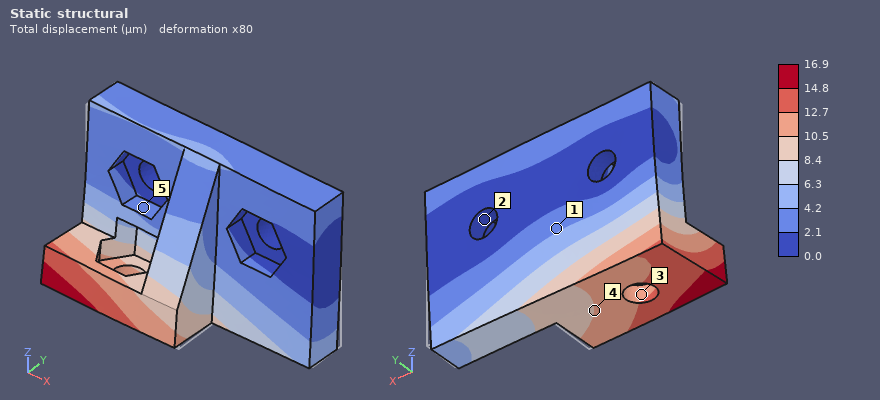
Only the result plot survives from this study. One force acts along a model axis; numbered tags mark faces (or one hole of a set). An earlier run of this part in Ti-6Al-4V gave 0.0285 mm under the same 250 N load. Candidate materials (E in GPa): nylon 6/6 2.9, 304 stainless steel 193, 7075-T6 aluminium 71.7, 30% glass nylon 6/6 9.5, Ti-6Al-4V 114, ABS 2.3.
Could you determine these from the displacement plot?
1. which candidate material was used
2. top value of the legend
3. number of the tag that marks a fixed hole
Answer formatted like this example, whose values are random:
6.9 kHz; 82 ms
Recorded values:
304 stainless steel; 16.9 µm; 2
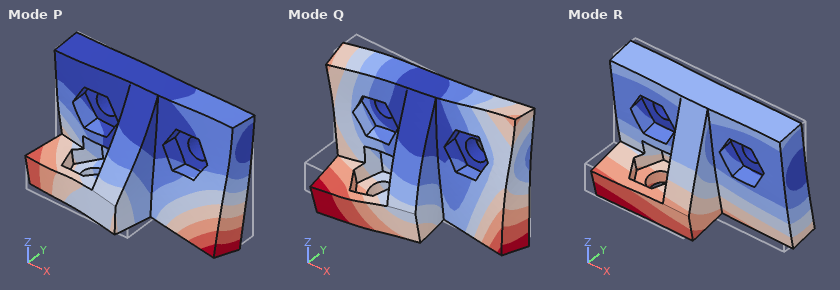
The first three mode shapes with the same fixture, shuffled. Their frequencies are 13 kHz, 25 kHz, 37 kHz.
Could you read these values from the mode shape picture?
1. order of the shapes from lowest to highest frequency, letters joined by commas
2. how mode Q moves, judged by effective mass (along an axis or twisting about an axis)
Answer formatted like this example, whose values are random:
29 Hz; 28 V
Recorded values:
R, P, Q; along X
